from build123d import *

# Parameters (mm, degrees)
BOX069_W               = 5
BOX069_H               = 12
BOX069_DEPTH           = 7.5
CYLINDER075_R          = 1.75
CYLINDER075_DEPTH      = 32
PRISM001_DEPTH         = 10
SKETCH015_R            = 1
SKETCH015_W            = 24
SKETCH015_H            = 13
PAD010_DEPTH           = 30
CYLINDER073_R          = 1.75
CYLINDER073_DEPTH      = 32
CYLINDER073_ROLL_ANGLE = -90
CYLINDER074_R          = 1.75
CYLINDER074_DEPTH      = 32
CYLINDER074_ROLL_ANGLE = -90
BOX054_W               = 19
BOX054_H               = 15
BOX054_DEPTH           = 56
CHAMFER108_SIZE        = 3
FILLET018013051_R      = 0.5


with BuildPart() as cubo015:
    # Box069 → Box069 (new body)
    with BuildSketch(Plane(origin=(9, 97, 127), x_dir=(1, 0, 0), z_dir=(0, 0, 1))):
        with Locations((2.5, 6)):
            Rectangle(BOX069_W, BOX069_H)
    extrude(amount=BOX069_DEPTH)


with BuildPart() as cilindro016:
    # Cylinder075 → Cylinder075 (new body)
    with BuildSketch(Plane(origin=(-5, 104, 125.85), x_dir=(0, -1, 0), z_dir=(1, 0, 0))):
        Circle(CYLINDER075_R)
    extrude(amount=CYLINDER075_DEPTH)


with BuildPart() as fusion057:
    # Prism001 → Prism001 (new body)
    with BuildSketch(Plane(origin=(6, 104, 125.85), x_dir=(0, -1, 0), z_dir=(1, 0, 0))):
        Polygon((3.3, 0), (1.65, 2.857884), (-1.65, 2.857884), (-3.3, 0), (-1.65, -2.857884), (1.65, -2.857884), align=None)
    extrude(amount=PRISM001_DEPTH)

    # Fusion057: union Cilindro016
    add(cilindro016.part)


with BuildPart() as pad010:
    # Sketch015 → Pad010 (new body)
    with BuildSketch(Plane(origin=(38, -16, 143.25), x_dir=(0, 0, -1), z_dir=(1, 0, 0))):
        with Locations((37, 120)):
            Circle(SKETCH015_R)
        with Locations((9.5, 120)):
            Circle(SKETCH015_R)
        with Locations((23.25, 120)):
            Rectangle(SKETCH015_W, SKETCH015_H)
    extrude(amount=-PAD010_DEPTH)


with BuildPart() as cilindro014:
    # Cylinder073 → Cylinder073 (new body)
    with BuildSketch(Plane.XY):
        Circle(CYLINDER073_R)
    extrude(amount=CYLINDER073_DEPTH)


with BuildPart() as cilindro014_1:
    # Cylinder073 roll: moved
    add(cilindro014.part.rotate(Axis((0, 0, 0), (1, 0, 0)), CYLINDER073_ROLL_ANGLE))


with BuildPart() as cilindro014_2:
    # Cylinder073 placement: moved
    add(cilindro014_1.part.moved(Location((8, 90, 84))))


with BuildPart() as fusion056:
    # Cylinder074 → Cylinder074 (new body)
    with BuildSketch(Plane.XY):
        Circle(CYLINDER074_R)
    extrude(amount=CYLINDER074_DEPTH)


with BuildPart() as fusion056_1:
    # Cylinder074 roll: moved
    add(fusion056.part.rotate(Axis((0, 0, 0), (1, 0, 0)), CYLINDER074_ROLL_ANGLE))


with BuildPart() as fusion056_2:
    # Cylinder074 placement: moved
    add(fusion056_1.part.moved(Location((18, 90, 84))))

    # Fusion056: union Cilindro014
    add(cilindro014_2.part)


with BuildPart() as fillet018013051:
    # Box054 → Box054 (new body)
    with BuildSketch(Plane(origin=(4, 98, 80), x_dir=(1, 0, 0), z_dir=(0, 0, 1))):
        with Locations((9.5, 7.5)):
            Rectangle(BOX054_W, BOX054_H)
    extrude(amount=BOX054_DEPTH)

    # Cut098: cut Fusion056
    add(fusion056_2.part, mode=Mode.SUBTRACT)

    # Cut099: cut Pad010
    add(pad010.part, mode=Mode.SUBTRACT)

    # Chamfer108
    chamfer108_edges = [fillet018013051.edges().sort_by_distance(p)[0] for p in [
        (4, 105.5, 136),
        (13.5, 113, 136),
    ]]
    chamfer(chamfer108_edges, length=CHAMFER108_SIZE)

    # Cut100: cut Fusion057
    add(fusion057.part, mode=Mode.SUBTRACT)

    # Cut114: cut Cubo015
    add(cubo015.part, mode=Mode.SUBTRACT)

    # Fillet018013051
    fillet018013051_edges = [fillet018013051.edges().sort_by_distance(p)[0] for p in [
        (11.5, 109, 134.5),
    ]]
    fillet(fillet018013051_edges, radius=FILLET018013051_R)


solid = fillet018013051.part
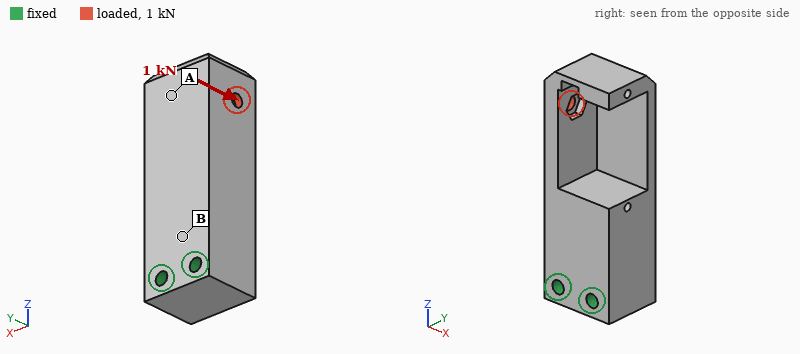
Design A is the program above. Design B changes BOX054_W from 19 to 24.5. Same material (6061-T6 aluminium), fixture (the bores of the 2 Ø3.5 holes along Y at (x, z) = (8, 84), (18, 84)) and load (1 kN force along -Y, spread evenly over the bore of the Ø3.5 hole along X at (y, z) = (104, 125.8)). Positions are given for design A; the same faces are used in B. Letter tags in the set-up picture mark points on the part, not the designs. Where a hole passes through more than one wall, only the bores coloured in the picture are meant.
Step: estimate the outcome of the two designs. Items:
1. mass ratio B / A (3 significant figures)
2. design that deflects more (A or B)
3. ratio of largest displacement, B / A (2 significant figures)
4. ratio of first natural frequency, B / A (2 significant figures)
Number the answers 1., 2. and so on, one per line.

1. 1.35
2. A
3. 0.74
4. 1.1
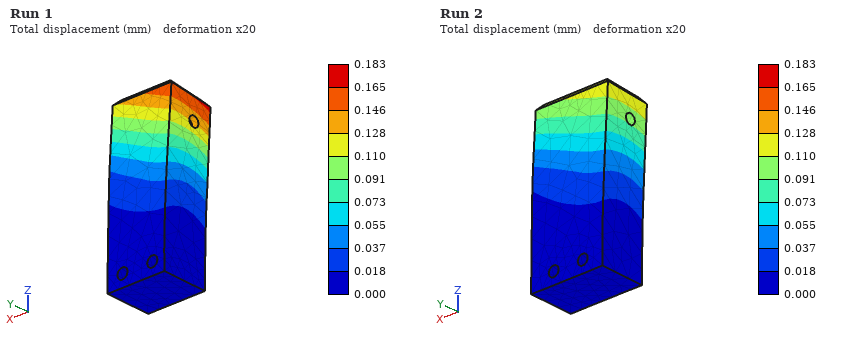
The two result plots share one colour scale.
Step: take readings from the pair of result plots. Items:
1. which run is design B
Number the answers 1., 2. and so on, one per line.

1. Run 2
